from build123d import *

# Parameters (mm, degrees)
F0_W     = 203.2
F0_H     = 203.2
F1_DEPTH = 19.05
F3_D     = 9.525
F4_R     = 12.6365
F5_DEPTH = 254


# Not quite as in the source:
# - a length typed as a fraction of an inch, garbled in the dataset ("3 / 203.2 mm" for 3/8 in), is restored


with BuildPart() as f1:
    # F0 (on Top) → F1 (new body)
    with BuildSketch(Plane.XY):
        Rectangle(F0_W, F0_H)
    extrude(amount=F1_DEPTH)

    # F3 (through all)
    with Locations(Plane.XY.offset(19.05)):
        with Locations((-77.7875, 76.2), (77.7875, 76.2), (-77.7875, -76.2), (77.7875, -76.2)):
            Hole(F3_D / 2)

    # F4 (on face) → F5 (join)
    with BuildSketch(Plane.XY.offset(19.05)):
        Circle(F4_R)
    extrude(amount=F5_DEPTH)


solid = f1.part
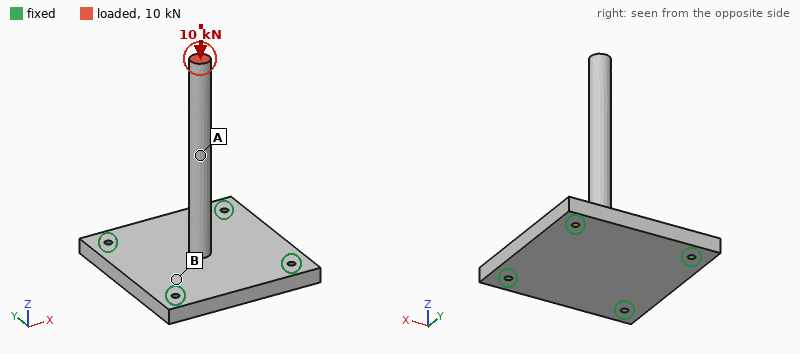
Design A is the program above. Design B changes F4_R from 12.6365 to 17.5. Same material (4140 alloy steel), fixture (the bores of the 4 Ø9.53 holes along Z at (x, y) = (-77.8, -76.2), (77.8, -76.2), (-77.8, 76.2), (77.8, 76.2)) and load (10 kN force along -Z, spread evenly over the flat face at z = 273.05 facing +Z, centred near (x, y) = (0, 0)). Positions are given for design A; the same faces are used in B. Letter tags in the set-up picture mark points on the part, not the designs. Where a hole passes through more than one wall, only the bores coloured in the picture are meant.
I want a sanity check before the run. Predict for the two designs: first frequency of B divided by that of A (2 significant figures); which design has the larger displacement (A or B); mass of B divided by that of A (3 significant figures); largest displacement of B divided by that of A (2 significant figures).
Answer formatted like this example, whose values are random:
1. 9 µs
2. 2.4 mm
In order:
1. 1.3
2. A
3. 1.13
4. 0.73
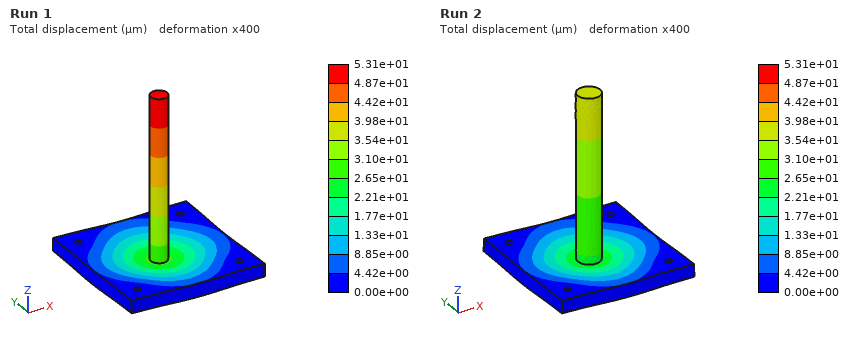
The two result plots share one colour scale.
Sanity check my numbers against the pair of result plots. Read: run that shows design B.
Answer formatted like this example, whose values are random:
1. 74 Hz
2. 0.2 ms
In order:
1. Run 2
